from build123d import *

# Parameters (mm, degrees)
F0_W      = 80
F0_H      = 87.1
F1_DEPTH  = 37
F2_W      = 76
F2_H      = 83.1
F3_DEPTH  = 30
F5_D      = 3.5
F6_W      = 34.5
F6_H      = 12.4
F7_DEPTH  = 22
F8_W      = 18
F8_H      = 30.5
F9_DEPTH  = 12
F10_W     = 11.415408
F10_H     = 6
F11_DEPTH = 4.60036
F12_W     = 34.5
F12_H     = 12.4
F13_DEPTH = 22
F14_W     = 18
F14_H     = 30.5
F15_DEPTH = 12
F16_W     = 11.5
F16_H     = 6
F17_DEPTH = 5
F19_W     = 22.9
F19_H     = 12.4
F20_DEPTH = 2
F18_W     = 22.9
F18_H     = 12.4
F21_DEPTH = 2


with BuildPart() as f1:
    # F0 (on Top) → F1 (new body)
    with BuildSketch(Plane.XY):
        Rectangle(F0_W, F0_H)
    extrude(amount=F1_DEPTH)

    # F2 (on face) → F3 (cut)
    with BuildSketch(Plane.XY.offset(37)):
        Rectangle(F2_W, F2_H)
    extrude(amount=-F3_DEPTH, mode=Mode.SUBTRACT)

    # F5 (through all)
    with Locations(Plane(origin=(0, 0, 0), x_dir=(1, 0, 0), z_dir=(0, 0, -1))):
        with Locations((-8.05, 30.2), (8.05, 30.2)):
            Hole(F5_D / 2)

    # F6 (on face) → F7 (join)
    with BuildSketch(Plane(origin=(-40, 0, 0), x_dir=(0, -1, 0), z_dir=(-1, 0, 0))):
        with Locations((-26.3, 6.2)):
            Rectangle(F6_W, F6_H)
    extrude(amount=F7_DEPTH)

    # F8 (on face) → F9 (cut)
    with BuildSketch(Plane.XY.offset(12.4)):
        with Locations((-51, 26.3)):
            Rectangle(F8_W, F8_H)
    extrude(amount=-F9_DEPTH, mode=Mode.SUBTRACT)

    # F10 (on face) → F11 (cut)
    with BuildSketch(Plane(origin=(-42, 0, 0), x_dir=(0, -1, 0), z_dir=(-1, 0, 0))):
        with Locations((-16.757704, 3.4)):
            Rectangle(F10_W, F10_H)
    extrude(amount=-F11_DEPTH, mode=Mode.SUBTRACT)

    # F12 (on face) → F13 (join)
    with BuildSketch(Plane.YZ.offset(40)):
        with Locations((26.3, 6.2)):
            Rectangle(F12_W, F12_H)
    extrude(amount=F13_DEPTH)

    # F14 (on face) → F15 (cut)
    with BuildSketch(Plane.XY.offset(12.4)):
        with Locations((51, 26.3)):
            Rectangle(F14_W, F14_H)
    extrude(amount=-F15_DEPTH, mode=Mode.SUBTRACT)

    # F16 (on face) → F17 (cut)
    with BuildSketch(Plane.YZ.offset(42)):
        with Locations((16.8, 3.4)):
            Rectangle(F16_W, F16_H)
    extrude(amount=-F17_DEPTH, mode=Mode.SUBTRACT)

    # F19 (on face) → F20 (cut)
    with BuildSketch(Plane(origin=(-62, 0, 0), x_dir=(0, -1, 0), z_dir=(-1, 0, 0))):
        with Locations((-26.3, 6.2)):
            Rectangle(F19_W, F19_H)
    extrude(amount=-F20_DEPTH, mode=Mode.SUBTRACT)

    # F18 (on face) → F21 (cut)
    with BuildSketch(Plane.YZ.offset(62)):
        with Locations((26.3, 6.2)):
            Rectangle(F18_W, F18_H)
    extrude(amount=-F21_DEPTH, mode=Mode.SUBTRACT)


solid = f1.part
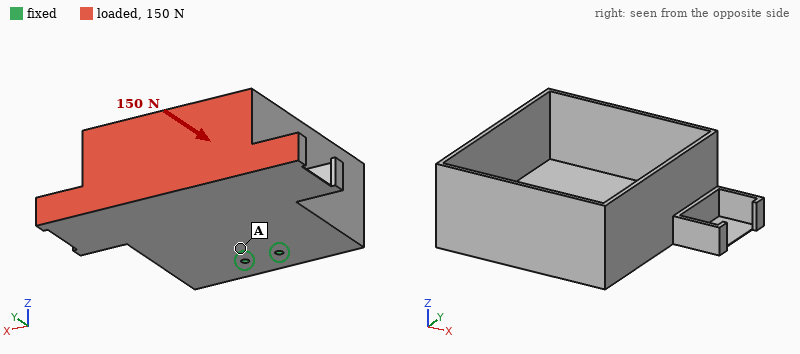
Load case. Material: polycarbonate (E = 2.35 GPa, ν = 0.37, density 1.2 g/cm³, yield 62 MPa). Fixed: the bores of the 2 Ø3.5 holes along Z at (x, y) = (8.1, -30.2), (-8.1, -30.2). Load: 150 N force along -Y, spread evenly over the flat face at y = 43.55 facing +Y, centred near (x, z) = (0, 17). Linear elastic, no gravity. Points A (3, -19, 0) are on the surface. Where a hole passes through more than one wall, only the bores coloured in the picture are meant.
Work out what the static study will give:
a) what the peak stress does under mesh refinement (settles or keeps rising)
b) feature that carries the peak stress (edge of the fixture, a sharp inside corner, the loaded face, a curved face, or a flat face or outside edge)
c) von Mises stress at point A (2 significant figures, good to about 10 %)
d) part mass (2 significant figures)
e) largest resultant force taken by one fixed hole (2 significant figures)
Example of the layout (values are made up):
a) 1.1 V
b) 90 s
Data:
a) keeps rising
b) edge of the fixture
c) 1.7 MPa
d) 86 g
e) 75 N
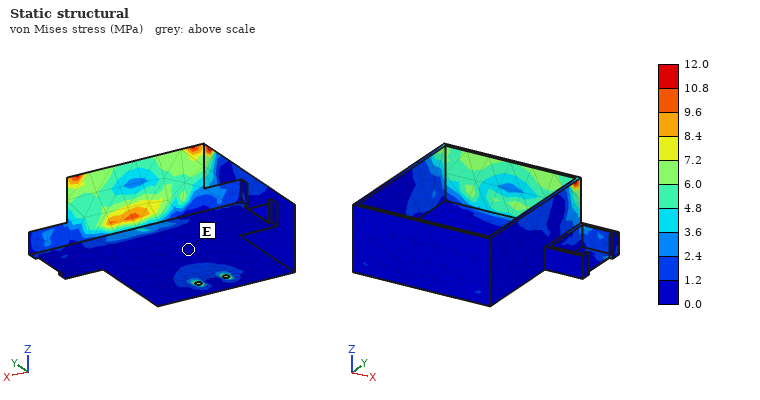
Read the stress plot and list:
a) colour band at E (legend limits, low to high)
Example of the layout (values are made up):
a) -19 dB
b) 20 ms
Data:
a) 0.0 to 1.2 MPa
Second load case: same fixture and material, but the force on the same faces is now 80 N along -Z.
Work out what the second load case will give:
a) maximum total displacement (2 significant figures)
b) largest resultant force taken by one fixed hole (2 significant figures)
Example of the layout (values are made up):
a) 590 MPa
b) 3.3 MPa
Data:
a) 1.7 mm
b) 43 N
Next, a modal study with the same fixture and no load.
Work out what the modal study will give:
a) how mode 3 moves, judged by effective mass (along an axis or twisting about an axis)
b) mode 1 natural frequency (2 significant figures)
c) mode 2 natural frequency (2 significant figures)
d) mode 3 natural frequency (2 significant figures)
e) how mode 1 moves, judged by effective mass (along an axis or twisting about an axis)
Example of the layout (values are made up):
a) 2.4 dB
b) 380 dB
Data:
a) along X
b) 220 Hz
c) 300 Hz
d) 550 Hz
e) along Z
